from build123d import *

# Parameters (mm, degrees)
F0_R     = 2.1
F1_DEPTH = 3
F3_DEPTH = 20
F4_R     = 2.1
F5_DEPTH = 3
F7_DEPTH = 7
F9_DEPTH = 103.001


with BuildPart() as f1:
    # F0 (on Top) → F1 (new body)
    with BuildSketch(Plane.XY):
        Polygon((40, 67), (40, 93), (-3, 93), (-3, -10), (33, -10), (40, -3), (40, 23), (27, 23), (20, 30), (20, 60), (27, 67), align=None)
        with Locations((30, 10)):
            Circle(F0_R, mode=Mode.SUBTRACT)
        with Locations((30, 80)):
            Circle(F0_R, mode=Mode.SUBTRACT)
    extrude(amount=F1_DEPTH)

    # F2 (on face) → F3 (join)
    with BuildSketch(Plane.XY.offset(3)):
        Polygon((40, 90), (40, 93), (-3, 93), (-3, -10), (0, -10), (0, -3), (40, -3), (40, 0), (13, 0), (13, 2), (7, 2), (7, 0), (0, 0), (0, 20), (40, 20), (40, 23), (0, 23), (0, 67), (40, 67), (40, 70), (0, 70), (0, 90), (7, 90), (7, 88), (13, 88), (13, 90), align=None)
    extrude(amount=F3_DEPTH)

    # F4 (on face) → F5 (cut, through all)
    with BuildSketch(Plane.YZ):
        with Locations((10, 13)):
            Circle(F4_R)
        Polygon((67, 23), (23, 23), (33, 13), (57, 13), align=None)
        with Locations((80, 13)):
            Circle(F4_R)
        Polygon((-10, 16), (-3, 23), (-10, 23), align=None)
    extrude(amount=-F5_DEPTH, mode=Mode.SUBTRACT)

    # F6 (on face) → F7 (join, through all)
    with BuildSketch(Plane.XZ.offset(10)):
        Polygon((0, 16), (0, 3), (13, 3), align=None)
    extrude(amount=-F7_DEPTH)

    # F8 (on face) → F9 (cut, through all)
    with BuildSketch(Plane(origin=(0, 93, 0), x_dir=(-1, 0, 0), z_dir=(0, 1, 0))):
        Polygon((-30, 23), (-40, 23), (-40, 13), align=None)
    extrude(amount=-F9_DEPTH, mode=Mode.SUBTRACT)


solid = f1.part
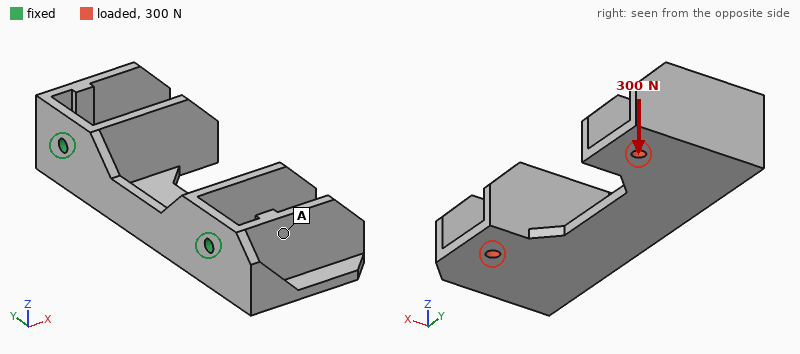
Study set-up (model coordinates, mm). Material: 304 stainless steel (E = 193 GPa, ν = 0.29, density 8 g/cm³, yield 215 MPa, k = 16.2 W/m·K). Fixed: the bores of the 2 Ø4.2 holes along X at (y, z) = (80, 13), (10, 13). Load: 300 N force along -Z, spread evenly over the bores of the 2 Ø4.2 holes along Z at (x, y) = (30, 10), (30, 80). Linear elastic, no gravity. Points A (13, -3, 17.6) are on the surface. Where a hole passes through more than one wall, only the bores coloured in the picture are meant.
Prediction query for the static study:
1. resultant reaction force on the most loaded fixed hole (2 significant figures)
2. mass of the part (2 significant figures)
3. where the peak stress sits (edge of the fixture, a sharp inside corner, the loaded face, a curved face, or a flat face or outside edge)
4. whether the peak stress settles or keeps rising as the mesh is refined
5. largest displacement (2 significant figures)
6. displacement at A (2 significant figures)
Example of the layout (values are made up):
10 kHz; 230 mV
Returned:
150 N; 210 g; edge of the fixture; keeps rising; 62 µm; 21 µm
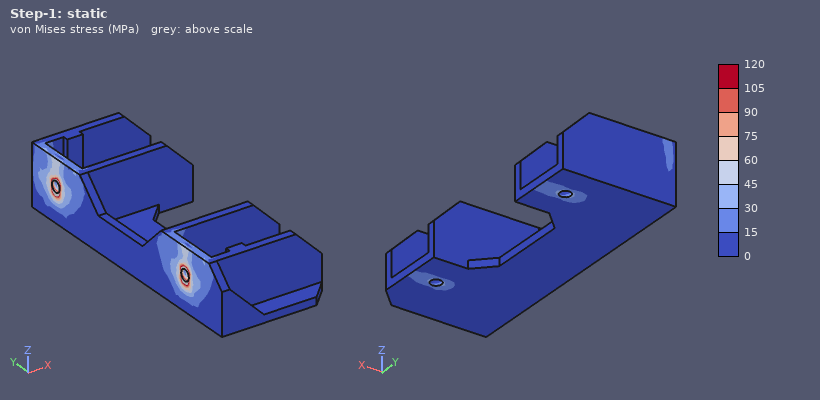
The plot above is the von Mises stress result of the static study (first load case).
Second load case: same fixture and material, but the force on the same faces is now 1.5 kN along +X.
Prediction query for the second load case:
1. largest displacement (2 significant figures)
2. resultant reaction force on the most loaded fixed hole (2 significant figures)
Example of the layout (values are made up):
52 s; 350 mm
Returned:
96 µm; 750 N
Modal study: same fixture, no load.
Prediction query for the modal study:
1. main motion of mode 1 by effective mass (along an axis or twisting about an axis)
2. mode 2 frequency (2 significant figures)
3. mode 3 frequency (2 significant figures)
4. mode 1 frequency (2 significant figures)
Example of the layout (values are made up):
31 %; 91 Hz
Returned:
along Z; 1600 Hz; 3200 Hz; 1400 Hz
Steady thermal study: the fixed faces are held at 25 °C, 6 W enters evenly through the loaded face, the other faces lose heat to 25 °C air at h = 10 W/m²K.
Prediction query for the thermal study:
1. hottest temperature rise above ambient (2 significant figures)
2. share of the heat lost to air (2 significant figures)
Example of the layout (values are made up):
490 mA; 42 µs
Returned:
47 K; 49 %
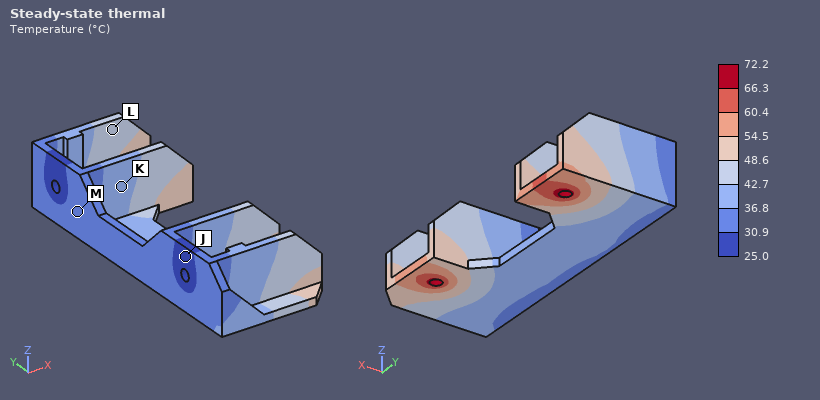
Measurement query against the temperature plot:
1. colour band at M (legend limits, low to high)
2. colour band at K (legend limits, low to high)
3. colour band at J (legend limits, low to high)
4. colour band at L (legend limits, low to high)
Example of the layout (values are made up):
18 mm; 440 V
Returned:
30.9 to 36.8 °C; 36.8 to 42.7 °C; 25.0 to 30.9 °C; 42.7 to 48.6 °C
